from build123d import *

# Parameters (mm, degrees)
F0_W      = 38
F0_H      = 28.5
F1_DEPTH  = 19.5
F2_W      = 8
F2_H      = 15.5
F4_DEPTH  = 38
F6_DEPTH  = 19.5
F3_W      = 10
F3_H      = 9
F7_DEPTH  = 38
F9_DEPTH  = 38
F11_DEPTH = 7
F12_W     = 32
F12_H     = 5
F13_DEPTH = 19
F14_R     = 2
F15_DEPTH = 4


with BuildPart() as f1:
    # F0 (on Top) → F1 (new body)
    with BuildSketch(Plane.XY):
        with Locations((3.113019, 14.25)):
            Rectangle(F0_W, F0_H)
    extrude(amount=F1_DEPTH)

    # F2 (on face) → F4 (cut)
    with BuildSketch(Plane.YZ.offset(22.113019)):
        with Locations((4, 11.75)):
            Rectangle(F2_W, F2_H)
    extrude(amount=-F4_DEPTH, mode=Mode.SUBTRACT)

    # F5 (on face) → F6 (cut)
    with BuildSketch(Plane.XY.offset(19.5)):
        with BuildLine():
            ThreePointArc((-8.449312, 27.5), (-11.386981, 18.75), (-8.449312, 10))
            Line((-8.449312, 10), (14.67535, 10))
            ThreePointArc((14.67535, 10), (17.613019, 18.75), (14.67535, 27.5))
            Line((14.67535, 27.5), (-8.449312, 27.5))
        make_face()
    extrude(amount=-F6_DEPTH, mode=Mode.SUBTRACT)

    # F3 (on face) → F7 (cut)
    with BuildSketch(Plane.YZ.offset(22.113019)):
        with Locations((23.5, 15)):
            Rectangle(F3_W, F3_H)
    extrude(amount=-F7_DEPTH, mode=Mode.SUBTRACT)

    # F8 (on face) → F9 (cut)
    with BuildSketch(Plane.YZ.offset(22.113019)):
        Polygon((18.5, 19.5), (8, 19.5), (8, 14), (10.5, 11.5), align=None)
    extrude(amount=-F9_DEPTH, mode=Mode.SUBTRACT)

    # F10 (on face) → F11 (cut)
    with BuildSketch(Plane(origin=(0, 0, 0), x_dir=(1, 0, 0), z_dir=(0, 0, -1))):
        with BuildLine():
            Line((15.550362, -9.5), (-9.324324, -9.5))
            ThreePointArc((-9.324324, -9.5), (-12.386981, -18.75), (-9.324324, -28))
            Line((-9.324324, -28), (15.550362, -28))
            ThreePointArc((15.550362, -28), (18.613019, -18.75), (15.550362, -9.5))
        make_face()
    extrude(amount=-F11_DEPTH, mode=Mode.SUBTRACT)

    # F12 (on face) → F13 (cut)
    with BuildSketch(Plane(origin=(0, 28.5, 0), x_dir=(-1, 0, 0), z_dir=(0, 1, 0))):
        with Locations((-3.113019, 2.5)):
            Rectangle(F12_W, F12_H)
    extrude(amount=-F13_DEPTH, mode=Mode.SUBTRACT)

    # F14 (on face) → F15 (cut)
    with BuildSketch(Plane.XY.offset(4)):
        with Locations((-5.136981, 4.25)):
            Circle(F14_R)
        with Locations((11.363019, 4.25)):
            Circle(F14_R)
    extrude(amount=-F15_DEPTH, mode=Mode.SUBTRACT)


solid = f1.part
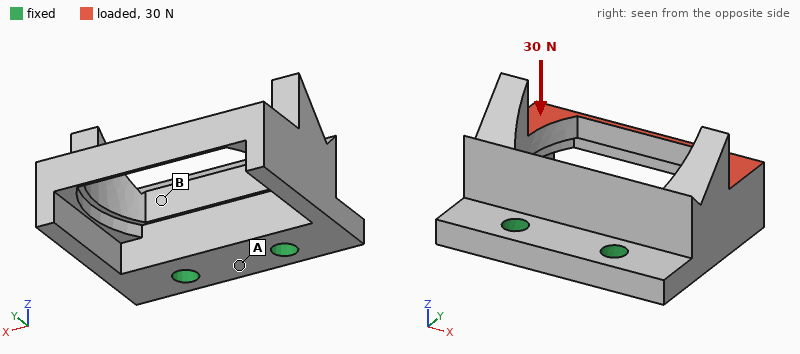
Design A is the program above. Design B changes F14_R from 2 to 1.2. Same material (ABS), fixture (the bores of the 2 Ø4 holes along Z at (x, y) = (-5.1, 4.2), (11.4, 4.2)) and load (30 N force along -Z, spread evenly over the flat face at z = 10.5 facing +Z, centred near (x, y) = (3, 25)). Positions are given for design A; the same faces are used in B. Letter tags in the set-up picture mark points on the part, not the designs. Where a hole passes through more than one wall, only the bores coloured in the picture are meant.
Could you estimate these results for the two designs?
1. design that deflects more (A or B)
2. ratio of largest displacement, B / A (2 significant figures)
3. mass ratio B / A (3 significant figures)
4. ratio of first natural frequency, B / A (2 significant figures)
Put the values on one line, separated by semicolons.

B; 1.1; 1.02; 0.94
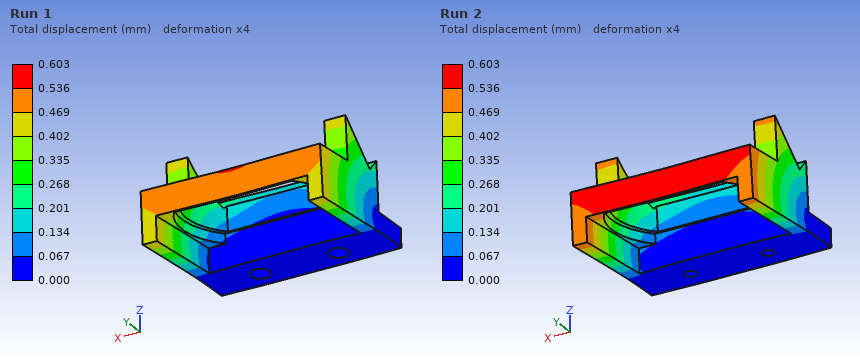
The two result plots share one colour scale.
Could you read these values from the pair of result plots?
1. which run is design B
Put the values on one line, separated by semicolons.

Run 2
